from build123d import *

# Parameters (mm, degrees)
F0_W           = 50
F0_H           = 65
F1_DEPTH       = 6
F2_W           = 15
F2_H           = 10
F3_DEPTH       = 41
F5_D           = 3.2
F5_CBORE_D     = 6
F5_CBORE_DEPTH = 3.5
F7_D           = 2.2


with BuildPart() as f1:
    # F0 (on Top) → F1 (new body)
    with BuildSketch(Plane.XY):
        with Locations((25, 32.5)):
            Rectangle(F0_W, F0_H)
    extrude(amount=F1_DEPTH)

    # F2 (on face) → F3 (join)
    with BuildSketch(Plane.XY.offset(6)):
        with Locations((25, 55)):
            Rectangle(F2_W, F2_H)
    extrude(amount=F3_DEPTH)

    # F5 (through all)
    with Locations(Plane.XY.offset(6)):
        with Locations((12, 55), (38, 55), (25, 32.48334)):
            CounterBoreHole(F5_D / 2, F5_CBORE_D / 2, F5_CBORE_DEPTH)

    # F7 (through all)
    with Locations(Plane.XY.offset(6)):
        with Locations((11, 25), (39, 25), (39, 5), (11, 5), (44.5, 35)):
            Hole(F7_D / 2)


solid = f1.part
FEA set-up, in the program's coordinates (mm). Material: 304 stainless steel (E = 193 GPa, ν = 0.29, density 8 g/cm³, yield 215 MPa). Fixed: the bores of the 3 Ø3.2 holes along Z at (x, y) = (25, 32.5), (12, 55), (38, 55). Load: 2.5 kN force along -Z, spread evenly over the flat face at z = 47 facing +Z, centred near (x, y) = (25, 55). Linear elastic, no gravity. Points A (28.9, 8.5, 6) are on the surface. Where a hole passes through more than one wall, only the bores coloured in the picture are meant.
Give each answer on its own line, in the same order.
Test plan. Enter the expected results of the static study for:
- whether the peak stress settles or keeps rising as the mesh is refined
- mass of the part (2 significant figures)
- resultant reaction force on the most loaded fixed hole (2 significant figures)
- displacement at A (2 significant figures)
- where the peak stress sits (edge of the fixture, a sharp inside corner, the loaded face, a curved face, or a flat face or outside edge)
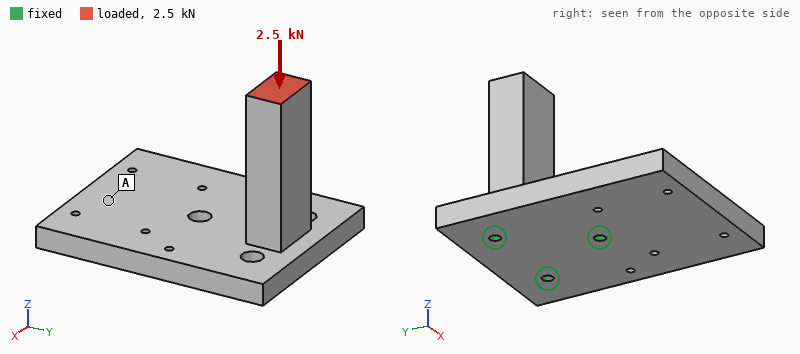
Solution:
keeps rising
200 g
1.4 kN
2.0 µm
edge of the fixture
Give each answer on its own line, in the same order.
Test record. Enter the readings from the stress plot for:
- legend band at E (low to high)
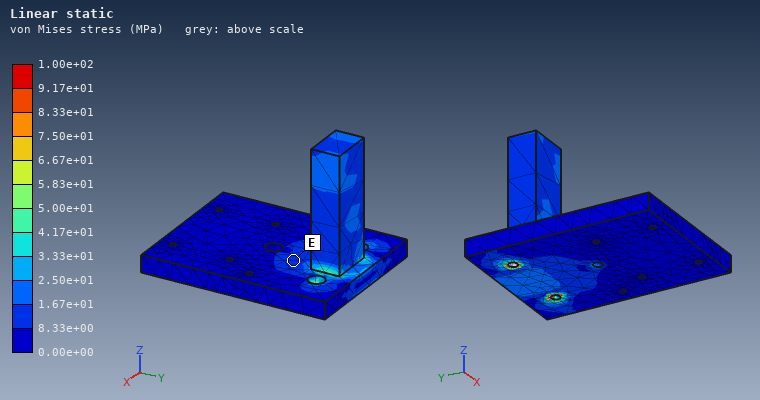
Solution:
8.33e+00 to 1.67e+01 MPa
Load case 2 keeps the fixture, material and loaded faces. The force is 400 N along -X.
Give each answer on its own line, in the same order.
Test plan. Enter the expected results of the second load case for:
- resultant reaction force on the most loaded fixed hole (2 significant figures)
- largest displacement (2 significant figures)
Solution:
760 N
30 µm
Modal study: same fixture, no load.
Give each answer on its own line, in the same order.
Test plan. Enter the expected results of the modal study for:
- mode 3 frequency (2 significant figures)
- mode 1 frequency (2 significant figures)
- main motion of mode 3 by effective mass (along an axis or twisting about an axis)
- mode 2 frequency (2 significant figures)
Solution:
3800 Hz
3000 Hz
twisting about Y
3000 Hz
